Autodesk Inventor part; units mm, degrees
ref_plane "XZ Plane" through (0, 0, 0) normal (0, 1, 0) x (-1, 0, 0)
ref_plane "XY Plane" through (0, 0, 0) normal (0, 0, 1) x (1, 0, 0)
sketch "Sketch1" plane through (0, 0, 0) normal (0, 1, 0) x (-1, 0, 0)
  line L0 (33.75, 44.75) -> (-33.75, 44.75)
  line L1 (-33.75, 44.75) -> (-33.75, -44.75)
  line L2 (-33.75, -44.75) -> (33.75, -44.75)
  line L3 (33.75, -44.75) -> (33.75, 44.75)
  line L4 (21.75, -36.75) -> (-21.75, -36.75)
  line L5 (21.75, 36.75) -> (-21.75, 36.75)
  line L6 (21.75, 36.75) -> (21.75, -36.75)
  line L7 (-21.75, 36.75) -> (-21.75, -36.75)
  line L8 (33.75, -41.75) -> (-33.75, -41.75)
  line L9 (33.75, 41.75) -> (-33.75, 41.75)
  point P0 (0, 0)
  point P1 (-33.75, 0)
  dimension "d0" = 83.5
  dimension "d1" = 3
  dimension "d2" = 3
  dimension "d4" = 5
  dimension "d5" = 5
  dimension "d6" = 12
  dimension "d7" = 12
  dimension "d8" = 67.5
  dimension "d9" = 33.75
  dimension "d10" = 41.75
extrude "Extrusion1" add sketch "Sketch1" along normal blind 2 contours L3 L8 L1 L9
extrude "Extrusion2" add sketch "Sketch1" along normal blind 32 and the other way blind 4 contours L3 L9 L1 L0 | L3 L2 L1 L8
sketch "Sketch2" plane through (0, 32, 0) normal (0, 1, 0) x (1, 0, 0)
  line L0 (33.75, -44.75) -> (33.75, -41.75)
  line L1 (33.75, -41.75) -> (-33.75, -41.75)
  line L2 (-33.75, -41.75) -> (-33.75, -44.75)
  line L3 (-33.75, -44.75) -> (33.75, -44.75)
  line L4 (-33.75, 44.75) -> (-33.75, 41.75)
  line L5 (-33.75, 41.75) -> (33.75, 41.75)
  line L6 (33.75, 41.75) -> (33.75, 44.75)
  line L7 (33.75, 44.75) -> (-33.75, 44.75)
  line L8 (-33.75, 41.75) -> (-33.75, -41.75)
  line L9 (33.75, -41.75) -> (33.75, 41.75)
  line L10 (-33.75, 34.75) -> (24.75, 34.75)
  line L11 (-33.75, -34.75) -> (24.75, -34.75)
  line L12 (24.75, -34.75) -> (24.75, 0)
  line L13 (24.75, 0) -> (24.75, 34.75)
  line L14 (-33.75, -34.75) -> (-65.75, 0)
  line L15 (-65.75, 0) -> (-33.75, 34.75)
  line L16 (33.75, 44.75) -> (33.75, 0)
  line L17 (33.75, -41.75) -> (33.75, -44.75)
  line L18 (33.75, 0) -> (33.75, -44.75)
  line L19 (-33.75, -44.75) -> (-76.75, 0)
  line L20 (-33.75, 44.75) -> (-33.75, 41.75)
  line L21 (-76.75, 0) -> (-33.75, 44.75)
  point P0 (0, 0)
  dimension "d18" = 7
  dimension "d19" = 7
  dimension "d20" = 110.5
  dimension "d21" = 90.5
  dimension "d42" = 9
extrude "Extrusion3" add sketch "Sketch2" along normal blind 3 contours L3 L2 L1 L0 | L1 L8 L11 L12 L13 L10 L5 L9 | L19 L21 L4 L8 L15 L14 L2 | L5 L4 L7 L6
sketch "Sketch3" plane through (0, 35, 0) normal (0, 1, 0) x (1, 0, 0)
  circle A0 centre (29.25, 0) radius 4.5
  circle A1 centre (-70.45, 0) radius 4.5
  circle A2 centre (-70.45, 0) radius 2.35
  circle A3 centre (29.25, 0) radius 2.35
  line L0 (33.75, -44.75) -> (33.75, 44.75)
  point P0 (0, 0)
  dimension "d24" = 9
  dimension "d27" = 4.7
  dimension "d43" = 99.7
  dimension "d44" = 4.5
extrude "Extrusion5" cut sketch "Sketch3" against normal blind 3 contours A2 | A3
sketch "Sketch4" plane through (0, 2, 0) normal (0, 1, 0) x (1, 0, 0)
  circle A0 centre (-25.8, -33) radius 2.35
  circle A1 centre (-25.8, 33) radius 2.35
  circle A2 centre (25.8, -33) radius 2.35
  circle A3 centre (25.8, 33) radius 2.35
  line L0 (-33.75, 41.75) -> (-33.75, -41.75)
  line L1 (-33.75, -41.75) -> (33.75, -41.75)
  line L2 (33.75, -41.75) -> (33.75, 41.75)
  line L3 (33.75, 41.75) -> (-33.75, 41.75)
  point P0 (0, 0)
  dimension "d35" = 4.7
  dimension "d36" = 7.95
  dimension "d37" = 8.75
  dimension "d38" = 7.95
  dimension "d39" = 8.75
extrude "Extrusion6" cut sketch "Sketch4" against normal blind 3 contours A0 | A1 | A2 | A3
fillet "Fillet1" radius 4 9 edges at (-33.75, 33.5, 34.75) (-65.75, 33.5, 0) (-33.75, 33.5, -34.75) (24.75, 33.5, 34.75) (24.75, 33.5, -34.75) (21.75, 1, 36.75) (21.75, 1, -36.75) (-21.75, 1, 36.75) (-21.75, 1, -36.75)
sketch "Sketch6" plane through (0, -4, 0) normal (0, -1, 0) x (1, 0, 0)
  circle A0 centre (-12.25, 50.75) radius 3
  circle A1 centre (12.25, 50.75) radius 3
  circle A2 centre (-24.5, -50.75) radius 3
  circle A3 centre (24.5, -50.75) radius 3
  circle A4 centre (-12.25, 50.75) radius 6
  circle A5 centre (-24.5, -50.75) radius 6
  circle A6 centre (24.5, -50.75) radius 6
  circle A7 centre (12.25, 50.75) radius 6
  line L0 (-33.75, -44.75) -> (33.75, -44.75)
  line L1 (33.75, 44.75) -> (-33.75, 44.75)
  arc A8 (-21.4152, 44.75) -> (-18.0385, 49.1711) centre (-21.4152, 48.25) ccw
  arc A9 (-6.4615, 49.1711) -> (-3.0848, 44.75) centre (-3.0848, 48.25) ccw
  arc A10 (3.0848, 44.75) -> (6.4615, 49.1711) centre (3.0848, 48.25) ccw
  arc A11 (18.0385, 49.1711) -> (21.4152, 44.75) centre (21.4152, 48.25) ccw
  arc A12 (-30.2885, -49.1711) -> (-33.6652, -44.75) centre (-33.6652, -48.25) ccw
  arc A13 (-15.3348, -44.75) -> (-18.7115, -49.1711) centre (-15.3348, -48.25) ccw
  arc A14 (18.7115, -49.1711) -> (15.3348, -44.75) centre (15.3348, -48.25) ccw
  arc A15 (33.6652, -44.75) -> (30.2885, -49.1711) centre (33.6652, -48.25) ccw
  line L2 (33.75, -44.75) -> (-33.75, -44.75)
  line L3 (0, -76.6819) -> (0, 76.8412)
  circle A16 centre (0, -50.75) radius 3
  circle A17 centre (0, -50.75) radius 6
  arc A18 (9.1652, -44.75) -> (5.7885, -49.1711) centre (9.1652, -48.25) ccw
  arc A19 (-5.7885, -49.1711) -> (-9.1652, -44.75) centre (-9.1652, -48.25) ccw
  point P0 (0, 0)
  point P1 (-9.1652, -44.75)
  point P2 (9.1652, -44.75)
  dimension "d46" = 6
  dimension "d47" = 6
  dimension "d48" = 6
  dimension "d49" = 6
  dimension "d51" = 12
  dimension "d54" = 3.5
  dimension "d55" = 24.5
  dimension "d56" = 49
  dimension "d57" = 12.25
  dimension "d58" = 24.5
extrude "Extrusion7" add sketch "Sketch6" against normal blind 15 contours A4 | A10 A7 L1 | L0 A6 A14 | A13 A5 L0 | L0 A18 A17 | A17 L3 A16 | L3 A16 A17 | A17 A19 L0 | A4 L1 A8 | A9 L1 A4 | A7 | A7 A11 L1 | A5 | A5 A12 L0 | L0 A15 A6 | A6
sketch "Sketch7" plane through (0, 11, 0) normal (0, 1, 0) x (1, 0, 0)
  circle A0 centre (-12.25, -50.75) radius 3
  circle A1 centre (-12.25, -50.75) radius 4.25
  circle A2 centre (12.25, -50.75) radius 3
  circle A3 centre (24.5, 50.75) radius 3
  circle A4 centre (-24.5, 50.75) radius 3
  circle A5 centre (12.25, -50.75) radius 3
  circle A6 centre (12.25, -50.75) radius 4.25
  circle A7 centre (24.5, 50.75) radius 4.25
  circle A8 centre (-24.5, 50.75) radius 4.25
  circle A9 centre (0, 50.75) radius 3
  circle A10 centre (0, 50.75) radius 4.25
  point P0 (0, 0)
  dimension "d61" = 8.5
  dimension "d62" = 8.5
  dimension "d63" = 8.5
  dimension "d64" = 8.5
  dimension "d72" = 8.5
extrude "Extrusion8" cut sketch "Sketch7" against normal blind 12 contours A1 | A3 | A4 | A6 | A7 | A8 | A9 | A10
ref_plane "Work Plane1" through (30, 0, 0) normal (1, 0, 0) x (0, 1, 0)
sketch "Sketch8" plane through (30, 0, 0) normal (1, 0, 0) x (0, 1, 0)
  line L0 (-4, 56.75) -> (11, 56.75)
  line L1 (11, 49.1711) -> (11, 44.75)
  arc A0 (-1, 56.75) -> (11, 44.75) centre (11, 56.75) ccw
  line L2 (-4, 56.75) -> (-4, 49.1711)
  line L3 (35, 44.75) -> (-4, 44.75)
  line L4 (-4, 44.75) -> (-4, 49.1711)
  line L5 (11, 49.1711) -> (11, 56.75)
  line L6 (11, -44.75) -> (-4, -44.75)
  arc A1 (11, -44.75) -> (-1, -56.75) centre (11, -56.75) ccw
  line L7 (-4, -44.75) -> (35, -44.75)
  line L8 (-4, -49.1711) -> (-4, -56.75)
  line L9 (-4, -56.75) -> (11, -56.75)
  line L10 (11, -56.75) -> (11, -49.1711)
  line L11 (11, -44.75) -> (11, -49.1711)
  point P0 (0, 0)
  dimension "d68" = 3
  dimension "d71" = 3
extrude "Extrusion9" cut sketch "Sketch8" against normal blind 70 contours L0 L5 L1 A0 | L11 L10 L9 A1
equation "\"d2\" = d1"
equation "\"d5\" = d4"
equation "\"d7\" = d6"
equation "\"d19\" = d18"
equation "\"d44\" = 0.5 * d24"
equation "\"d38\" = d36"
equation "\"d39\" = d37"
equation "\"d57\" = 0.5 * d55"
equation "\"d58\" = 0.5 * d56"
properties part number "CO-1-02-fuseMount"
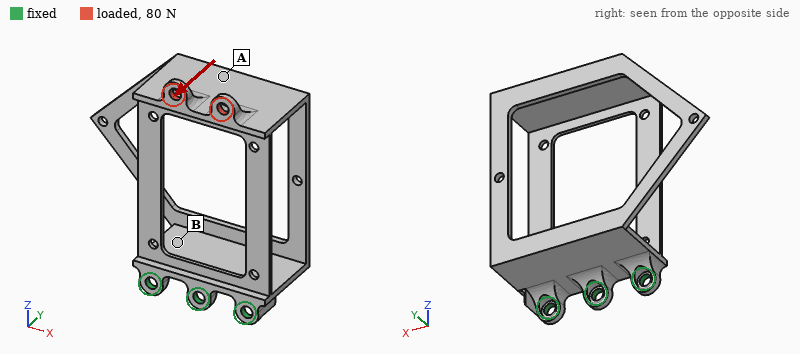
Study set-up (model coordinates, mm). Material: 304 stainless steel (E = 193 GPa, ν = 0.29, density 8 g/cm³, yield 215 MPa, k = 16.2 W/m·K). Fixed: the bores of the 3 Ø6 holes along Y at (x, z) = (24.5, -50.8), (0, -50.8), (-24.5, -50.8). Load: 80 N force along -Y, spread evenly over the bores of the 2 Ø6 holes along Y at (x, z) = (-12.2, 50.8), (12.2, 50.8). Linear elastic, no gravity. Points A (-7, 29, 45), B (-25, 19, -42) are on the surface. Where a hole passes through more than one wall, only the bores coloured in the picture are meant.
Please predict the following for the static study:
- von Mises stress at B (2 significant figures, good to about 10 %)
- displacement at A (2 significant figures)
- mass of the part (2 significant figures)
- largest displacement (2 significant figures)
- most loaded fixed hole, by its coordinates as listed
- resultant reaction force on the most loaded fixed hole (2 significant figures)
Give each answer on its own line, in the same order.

32 MPa
0.73 mm
250 g
0.77 mm
(0, -50.8)
81 N
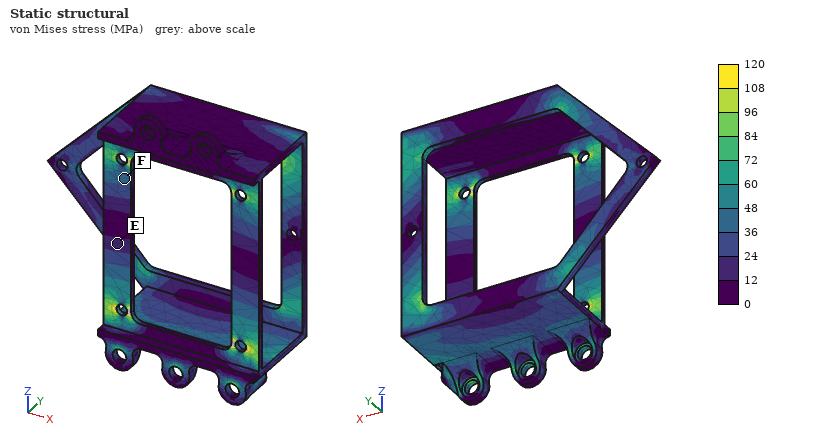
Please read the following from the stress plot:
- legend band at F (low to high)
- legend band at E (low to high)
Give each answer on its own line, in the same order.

36 to 48 MPa
12 to 24 MPa
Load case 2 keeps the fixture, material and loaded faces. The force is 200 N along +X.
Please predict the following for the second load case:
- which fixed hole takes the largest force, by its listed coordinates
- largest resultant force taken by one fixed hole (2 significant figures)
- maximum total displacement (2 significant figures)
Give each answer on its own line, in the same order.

(0, -50.8)
360 N
0.17 mm
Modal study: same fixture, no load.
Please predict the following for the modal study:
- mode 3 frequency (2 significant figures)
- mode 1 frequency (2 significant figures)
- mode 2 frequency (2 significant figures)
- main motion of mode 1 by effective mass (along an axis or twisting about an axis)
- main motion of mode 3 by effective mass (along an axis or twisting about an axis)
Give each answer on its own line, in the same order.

700 Hz
160 Hz
460 Hz
along Y
along X
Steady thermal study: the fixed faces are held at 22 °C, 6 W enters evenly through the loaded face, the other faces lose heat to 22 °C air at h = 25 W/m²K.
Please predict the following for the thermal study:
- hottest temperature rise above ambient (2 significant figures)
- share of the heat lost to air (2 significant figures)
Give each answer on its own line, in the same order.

73 K
99 %
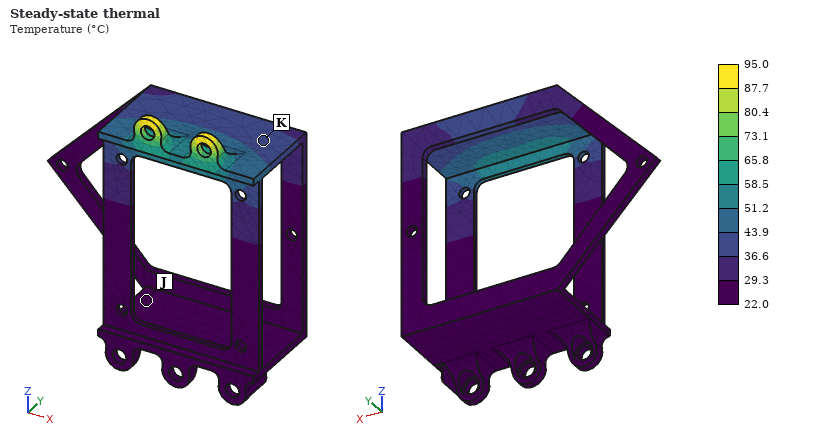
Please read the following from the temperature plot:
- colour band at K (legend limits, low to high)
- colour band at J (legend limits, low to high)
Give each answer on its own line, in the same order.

36.6 to 43.9 °C
22.0 to 29.3 °C
